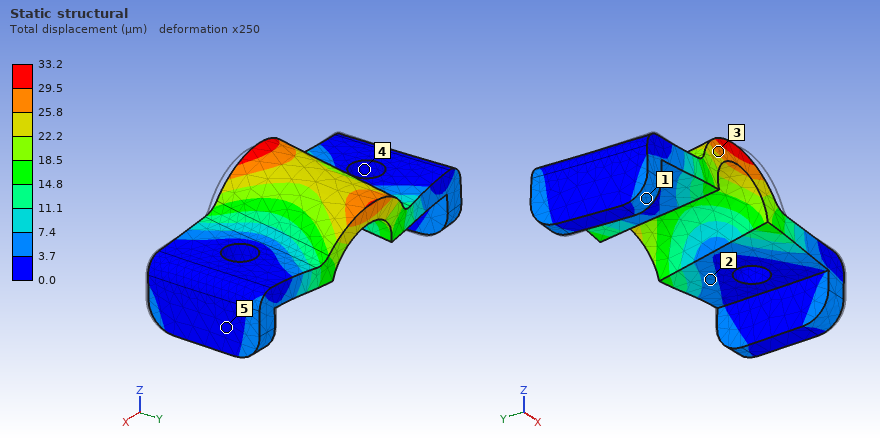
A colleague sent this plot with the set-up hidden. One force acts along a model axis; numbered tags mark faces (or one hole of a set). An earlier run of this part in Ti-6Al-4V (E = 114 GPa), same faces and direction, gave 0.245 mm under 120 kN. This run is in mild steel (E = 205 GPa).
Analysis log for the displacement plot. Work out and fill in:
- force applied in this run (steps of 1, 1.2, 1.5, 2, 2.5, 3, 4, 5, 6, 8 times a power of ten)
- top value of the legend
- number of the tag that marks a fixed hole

30 kN
33.2 µm
4
